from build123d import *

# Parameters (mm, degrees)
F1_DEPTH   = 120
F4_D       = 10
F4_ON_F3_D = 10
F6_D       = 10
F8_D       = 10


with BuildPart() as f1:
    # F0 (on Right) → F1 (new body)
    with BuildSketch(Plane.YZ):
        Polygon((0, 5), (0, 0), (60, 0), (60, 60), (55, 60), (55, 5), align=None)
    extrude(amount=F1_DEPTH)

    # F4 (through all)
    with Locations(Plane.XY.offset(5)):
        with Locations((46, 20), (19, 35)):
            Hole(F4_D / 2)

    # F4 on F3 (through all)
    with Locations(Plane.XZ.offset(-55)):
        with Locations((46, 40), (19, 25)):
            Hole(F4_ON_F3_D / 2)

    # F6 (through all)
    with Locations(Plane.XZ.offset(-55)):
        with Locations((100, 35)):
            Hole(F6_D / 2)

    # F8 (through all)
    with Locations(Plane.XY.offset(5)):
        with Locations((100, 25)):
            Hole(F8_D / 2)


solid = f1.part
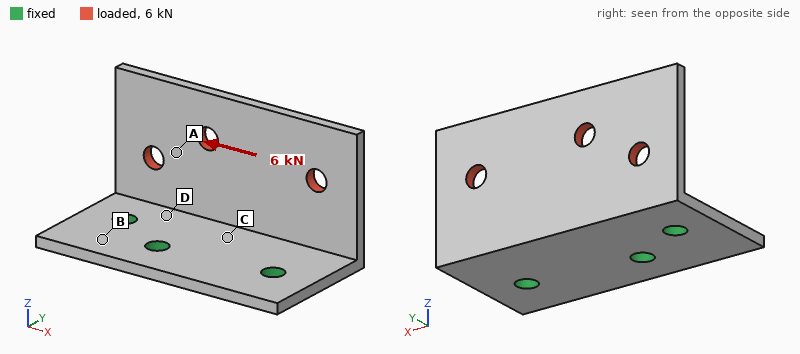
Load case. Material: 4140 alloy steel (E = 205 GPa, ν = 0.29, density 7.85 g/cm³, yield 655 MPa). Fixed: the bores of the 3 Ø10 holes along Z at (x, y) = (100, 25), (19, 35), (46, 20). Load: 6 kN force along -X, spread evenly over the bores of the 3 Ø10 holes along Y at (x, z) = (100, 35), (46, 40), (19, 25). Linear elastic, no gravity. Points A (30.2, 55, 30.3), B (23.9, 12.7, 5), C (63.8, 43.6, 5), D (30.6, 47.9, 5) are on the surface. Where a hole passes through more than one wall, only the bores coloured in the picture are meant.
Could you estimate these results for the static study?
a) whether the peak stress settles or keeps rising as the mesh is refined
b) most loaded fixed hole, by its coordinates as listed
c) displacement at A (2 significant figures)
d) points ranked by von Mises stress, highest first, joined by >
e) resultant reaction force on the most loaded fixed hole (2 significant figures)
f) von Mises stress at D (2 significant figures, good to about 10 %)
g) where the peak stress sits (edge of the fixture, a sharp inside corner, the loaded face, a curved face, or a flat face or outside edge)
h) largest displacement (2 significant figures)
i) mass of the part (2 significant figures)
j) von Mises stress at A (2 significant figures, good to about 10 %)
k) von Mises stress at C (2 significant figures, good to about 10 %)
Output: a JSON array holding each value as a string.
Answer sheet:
["keeps rising", "(19, 35)", "0.073 mm", "D > C > A > B", "4.1 kN", "110 MPa", "edge of the fixture", "0.33 mm", "520 g", "42 MPa", "70 MPa"]
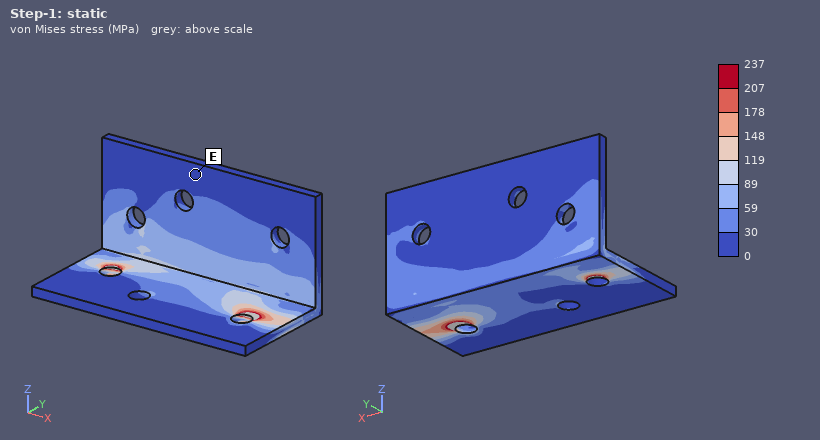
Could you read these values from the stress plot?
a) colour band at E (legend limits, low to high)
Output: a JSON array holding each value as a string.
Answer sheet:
["0 to 30 MPa"]
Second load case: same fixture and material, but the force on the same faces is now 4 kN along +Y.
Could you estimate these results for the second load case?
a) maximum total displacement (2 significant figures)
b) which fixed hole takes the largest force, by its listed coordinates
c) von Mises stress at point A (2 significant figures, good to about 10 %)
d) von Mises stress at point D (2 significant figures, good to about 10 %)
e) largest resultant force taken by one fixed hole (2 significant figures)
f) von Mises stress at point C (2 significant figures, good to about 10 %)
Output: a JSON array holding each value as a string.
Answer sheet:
["1.0 mm", "(46, 20)", "40 MPa", "260 MPa", "1.9 kN", "190 MPa"]
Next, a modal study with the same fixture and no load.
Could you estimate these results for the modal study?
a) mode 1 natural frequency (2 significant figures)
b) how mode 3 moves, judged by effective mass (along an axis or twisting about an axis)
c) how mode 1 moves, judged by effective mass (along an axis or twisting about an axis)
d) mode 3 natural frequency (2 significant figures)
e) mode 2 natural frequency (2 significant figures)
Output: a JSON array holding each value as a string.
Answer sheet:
["740 Hz", "along Z", "along Y", "2100 Hz", "1400 Hz"]
